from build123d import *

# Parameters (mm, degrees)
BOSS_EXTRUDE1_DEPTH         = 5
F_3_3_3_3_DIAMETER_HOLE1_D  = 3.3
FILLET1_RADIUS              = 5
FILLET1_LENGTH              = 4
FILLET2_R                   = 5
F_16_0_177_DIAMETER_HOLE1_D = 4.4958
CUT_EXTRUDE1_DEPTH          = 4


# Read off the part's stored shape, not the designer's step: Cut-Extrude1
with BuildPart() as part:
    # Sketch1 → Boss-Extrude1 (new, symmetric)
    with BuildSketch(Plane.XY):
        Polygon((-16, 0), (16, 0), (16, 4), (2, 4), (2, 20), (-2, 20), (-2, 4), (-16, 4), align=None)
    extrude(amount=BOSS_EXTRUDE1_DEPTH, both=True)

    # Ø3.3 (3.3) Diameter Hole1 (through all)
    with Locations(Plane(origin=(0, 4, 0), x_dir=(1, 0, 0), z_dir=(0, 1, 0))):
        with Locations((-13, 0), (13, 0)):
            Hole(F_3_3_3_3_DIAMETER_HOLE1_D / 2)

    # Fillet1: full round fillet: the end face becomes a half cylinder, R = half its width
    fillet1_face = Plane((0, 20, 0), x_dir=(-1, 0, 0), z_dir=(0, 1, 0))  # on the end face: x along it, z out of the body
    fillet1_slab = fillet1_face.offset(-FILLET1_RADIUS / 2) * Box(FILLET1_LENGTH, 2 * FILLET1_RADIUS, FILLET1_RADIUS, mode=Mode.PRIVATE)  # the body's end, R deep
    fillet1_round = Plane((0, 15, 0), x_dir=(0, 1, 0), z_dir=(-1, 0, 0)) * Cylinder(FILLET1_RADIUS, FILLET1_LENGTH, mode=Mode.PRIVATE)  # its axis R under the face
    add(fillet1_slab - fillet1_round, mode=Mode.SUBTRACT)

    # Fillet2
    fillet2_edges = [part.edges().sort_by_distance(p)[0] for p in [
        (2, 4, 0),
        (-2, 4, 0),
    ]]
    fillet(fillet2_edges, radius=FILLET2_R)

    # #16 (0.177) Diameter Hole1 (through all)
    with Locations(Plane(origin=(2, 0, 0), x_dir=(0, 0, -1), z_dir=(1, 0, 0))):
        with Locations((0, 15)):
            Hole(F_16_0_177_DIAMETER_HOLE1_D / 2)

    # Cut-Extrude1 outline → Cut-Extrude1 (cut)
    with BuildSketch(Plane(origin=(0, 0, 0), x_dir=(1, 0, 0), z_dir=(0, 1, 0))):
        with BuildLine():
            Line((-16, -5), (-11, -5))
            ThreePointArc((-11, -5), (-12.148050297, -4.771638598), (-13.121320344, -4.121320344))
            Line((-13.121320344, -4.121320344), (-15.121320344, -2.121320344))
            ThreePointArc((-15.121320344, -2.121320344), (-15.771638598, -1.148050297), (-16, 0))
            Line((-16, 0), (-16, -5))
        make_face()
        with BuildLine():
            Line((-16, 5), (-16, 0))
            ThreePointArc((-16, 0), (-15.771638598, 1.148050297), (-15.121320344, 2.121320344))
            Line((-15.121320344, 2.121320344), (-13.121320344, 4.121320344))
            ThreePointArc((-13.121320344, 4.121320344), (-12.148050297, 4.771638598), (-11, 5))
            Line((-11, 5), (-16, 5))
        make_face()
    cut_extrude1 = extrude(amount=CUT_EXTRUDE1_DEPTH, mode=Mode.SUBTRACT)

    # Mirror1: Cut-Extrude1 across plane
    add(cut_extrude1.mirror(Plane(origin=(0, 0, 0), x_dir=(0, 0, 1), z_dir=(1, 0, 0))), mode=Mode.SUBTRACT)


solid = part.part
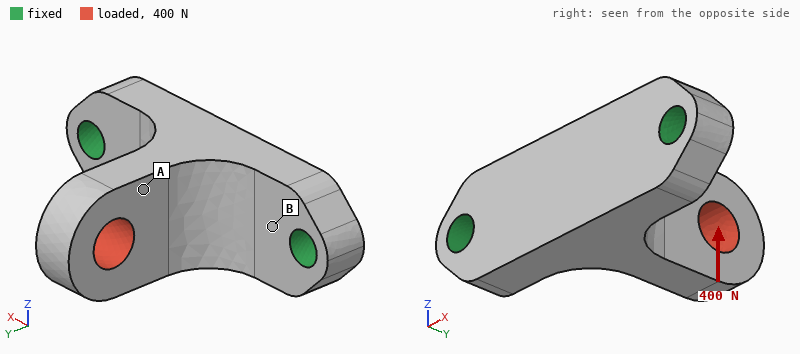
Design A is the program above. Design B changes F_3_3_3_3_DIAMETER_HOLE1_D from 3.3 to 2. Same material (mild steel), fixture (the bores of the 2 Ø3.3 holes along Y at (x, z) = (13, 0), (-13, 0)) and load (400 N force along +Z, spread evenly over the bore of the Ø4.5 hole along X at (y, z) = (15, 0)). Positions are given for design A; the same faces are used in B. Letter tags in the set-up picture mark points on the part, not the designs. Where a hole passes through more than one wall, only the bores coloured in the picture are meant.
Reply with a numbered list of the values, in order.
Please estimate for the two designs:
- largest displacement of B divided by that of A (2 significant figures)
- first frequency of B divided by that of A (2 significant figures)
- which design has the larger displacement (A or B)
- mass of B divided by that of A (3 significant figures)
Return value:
1. 1.2
2. 0.91
3. B
4. 1.02
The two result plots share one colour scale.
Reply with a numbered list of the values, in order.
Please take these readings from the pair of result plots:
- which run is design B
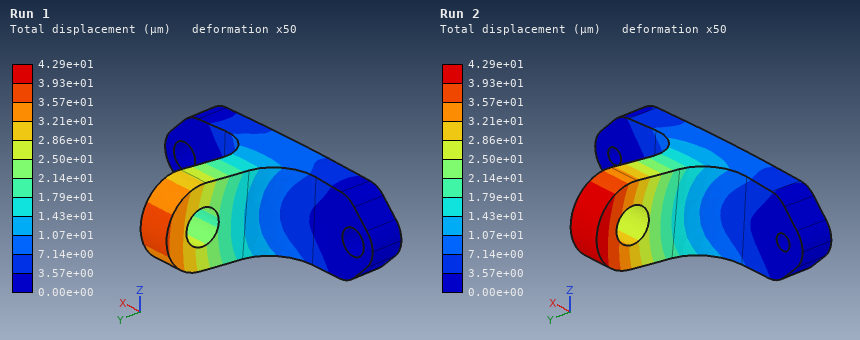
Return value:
1. Run 2
